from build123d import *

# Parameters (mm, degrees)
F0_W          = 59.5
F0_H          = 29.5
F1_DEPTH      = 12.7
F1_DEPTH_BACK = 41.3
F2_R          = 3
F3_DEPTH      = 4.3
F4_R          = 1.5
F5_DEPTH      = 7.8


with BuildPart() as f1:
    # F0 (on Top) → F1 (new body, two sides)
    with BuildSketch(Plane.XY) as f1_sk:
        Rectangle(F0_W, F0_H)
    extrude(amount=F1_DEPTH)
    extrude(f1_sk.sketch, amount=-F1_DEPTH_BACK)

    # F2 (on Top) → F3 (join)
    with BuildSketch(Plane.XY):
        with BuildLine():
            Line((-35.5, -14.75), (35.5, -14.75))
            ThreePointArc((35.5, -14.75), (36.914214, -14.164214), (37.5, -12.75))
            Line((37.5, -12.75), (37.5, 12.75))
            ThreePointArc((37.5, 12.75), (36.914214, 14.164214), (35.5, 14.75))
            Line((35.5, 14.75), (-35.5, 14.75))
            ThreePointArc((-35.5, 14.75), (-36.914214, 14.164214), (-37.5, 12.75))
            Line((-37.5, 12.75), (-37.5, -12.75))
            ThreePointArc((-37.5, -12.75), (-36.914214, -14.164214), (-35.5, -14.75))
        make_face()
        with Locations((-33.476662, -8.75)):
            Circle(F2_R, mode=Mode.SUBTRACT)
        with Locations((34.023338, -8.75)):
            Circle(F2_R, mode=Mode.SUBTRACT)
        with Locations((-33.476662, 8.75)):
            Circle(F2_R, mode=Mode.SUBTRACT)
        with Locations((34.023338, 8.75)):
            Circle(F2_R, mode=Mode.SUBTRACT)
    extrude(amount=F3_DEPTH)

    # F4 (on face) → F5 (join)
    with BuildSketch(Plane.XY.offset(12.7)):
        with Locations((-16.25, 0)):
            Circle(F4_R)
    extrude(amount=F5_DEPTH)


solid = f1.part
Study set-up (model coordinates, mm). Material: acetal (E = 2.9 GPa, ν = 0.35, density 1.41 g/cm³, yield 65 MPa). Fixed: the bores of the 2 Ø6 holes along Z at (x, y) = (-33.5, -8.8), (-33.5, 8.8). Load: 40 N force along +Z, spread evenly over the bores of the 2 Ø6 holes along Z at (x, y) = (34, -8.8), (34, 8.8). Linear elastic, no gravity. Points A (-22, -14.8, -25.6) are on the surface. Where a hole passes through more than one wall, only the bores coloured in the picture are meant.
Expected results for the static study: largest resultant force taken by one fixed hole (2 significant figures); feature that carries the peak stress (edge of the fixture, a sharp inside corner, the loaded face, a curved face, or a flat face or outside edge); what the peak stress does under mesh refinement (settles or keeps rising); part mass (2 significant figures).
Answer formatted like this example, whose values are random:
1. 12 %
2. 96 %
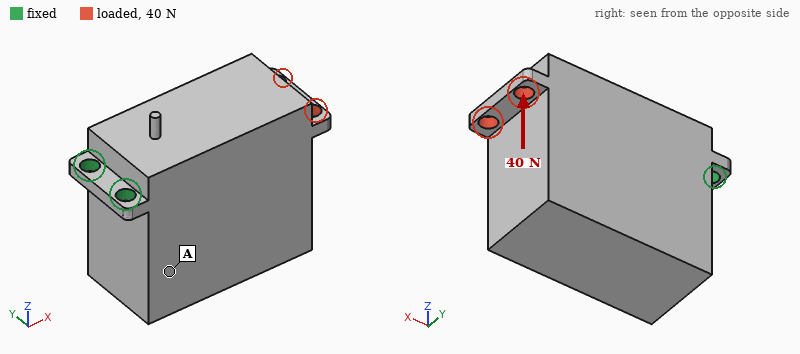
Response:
1. 20 N
2. edge of the fixture
3. keeps rising
4. 140 g
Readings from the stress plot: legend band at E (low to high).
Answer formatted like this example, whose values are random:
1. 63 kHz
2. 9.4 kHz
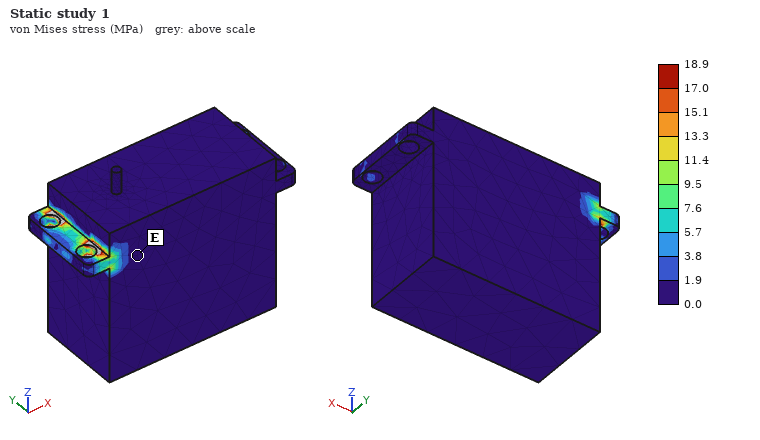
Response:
1. 0.0 to 1.9 MPa
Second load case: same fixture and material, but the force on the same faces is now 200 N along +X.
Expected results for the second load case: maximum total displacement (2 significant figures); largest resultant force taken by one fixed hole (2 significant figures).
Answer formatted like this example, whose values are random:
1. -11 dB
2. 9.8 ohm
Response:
1. 39 µm
2. 100 N
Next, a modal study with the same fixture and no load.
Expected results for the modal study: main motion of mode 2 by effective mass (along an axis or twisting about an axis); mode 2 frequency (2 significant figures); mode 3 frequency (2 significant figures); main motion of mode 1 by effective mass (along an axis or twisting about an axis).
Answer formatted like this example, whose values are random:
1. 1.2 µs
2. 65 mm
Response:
1. along Y
2. 570 Hz
3. 1000 Hz
4. along Z
